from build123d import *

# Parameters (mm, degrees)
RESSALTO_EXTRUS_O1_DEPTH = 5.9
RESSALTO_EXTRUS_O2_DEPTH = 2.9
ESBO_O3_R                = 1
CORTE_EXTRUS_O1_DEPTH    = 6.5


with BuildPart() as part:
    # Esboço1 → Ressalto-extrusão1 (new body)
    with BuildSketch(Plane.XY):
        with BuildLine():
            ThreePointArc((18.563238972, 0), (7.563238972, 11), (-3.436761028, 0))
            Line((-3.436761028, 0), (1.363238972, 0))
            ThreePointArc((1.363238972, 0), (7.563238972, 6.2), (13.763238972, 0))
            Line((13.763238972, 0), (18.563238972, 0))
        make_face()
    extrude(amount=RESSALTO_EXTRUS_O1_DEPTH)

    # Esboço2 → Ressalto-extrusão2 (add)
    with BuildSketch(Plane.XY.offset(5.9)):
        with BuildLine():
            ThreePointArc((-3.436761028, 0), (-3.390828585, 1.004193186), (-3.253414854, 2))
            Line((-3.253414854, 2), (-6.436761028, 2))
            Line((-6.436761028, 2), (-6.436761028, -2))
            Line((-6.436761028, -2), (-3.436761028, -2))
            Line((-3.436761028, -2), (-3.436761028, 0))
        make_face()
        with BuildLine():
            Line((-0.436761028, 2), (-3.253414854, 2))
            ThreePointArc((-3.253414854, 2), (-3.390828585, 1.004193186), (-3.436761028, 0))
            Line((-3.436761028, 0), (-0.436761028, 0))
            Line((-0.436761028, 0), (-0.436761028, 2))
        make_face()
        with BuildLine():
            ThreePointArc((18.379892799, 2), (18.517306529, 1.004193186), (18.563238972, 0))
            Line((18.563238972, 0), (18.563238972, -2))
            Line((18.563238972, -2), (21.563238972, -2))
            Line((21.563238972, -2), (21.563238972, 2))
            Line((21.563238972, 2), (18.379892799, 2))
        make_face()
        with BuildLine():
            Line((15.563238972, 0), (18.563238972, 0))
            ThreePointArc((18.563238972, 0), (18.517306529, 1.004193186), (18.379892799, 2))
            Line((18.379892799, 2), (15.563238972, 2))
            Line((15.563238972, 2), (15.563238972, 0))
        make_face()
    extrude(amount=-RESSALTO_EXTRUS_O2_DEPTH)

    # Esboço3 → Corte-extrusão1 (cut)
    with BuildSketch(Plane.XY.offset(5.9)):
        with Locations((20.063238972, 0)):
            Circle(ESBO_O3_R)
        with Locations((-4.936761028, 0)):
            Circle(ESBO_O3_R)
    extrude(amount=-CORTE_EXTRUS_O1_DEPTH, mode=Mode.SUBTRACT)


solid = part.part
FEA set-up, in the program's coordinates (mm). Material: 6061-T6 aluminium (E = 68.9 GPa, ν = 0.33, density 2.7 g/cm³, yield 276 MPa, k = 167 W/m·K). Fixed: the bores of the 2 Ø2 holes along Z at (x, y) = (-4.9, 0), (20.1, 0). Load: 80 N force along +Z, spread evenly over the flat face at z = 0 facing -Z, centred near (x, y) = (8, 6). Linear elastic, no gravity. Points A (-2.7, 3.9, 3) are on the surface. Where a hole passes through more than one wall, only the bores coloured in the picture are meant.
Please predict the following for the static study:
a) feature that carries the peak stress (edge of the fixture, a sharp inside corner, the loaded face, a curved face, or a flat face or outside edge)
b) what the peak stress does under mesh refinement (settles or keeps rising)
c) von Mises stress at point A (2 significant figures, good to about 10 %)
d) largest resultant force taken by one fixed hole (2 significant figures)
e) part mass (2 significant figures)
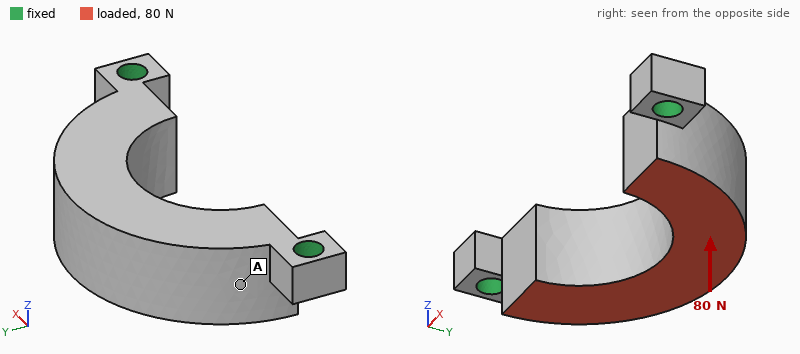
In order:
a sharp inside corner
keeps rising
10 MPa
40 N
2.2 g
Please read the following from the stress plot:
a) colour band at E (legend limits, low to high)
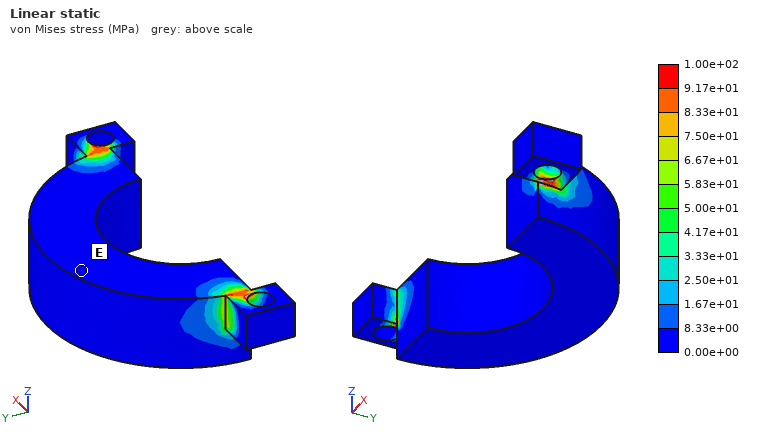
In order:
0.00e+00 to 8.33e+00 MPa
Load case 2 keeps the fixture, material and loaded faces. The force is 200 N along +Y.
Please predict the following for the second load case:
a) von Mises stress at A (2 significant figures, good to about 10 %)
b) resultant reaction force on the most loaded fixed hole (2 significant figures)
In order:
23 MPa
120 N
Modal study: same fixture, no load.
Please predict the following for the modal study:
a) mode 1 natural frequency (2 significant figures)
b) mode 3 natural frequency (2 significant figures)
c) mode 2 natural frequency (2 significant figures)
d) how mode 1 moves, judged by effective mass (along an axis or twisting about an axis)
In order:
7600 Hz
35 kHz
34 kHz
along Z
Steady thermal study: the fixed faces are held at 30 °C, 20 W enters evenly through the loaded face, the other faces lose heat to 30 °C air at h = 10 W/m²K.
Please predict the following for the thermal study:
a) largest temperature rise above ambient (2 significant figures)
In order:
36 K
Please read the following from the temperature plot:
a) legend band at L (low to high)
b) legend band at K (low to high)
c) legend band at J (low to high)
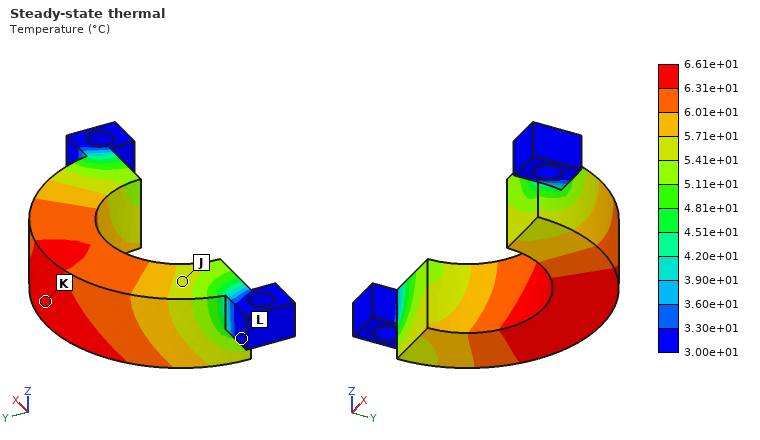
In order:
3.00e+01 to 3.30e+01 °C
6.31e+01 to 6.61e+01 °C
5.41e+01 to 5.71e+01 °C
